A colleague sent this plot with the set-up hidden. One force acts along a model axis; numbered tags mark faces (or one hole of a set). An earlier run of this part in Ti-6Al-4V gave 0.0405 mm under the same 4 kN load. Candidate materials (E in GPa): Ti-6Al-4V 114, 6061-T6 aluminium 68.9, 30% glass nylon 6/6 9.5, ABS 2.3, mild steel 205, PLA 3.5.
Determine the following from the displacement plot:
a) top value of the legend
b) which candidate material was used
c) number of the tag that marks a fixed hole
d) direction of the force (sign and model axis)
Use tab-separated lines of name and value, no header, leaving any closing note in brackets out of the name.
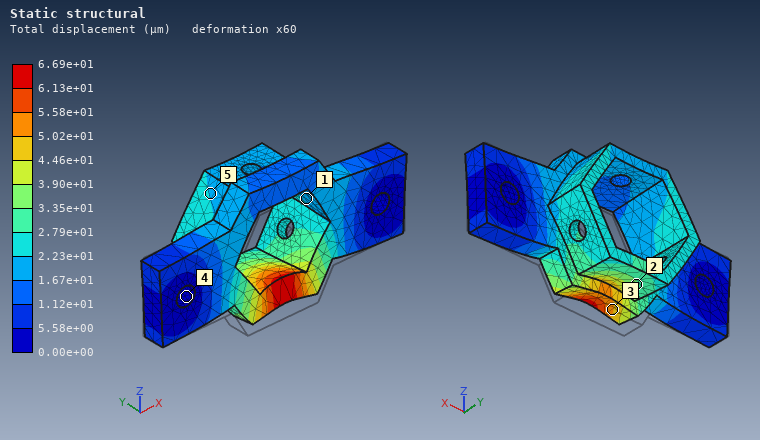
top value of the legend	6.69e+01 µm
which candidate material was used	6061-T6 aluminium
number of the tag that marks a fixed hole	4
direction of the force	+Z
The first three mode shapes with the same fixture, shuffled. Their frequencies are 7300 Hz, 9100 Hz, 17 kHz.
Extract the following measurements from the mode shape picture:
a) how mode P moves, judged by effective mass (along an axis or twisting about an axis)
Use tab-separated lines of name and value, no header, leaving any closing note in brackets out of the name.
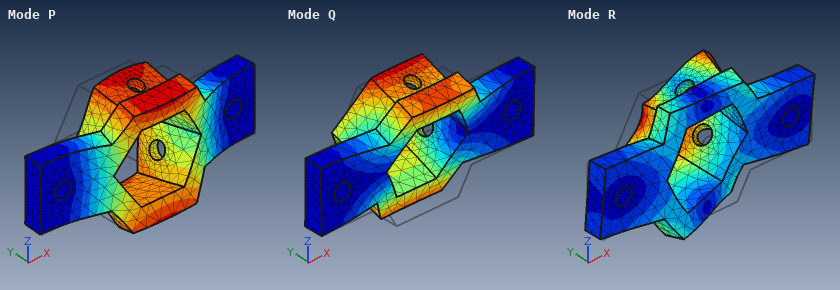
how mode P moves, judged by effective mass	along Y
